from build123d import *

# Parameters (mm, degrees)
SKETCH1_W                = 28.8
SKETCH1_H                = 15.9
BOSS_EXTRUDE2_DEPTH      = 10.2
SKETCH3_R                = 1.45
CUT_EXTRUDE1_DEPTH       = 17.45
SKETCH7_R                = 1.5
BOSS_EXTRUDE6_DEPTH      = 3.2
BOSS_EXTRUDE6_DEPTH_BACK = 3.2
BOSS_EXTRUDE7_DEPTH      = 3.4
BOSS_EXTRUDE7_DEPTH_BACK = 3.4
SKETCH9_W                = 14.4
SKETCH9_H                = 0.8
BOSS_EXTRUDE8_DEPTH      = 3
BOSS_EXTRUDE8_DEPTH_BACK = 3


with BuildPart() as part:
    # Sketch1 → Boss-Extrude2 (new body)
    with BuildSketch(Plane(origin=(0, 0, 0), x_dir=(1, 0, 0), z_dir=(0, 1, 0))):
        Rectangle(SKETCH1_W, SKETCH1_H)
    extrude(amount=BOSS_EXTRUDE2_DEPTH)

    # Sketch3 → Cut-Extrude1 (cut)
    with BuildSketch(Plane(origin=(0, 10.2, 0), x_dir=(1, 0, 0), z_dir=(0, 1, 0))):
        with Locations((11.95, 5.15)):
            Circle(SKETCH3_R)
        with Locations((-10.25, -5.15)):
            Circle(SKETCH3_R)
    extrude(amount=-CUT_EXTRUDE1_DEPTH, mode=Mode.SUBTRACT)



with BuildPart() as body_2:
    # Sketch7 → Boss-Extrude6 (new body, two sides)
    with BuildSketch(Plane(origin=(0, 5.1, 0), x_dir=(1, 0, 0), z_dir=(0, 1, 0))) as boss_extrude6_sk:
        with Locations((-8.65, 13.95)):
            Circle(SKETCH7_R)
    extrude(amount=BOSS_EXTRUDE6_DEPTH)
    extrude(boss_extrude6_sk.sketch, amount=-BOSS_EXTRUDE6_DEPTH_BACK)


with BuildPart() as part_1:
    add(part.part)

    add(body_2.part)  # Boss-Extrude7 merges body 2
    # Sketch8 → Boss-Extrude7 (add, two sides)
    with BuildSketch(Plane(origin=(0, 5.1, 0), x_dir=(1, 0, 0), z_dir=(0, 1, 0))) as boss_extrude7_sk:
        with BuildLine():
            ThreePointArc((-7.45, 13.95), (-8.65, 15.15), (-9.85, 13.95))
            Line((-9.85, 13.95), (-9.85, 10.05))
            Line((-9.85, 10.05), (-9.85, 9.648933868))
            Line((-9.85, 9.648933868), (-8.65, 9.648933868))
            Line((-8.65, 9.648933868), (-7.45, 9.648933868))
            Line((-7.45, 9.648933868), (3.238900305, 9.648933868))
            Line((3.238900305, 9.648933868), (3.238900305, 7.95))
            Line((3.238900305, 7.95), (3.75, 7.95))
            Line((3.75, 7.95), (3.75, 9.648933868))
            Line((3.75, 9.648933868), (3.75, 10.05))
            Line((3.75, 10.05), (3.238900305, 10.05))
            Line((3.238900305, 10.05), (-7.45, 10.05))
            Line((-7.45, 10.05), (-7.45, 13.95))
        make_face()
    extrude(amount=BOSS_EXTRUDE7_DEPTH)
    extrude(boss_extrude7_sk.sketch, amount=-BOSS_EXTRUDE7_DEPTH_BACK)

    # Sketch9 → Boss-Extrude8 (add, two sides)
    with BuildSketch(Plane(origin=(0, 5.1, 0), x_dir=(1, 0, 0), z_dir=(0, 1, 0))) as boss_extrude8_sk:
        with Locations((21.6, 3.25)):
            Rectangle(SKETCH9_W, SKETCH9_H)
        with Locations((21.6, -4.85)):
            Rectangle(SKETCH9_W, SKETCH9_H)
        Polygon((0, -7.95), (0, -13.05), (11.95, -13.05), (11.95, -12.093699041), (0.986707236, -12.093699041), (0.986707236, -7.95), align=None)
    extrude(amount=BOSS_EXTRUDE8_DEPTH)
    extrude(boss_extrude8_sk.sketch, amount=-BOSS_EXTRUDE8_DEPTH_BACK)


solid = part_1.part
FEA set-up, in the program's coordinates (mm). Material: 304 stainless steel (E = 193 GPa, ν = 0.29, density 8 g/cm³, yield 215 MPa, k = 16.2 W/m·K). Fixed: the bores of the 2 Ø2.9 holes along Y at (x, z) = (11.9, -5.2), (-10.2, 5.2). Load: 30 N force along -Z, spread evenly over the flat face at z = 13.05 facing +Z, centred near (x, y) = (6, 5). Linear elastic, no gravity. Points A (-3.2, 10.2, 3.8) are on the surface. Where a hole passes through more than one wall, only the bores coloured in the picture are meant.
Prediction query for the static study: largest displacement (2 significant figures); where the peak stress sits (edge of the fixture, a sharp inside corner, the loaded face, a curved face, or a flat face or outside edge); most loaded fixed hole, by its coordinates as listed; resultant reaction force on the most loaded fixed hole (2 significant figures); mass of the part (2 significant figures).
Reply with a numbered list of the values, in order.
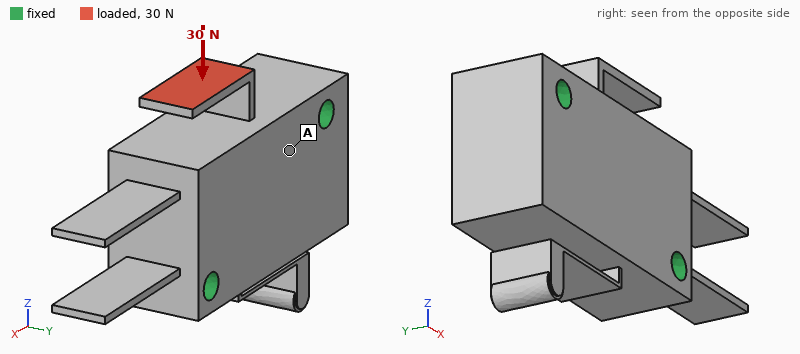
1. 0.15 mm
2. a flat face or outside edge
3. (11.9, -5.2)
4. 23 N
5. 39 g
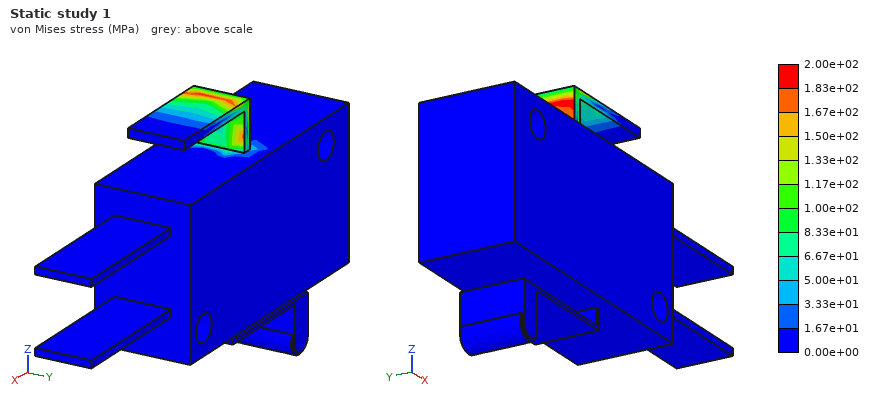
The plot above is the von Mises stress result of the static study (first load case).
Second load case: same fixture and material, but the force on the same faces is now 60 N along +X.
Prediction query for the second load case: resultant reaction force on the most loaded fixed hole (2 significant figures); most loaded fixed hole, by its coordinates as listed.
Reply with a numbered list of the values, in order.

1. 51 N
2. (-10.2, 5.2)
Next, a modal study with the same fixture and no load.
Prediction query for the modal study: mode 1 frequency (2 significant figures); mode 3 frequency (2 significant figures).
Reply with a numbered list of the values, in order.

1. 540 Hz
2. 3000 Hz
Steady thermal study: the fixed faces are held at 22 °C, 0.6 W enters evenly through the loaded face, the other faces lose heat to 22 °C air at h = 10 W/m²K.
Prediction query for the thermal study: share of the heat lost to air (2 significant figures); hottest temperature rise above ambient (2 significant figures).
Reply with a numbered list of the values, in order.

1. 13 %
2. 61 K
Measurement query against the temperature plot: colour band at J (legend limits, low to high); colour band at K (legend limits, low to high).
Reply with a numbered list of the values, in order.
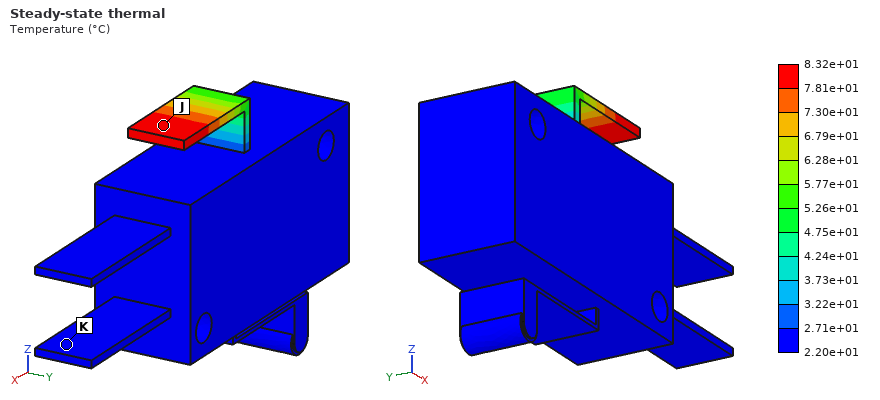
1. 7.81e+01 to 8.32e+01 °C
2. 2.20e+01 to 2.71e+01 °C
